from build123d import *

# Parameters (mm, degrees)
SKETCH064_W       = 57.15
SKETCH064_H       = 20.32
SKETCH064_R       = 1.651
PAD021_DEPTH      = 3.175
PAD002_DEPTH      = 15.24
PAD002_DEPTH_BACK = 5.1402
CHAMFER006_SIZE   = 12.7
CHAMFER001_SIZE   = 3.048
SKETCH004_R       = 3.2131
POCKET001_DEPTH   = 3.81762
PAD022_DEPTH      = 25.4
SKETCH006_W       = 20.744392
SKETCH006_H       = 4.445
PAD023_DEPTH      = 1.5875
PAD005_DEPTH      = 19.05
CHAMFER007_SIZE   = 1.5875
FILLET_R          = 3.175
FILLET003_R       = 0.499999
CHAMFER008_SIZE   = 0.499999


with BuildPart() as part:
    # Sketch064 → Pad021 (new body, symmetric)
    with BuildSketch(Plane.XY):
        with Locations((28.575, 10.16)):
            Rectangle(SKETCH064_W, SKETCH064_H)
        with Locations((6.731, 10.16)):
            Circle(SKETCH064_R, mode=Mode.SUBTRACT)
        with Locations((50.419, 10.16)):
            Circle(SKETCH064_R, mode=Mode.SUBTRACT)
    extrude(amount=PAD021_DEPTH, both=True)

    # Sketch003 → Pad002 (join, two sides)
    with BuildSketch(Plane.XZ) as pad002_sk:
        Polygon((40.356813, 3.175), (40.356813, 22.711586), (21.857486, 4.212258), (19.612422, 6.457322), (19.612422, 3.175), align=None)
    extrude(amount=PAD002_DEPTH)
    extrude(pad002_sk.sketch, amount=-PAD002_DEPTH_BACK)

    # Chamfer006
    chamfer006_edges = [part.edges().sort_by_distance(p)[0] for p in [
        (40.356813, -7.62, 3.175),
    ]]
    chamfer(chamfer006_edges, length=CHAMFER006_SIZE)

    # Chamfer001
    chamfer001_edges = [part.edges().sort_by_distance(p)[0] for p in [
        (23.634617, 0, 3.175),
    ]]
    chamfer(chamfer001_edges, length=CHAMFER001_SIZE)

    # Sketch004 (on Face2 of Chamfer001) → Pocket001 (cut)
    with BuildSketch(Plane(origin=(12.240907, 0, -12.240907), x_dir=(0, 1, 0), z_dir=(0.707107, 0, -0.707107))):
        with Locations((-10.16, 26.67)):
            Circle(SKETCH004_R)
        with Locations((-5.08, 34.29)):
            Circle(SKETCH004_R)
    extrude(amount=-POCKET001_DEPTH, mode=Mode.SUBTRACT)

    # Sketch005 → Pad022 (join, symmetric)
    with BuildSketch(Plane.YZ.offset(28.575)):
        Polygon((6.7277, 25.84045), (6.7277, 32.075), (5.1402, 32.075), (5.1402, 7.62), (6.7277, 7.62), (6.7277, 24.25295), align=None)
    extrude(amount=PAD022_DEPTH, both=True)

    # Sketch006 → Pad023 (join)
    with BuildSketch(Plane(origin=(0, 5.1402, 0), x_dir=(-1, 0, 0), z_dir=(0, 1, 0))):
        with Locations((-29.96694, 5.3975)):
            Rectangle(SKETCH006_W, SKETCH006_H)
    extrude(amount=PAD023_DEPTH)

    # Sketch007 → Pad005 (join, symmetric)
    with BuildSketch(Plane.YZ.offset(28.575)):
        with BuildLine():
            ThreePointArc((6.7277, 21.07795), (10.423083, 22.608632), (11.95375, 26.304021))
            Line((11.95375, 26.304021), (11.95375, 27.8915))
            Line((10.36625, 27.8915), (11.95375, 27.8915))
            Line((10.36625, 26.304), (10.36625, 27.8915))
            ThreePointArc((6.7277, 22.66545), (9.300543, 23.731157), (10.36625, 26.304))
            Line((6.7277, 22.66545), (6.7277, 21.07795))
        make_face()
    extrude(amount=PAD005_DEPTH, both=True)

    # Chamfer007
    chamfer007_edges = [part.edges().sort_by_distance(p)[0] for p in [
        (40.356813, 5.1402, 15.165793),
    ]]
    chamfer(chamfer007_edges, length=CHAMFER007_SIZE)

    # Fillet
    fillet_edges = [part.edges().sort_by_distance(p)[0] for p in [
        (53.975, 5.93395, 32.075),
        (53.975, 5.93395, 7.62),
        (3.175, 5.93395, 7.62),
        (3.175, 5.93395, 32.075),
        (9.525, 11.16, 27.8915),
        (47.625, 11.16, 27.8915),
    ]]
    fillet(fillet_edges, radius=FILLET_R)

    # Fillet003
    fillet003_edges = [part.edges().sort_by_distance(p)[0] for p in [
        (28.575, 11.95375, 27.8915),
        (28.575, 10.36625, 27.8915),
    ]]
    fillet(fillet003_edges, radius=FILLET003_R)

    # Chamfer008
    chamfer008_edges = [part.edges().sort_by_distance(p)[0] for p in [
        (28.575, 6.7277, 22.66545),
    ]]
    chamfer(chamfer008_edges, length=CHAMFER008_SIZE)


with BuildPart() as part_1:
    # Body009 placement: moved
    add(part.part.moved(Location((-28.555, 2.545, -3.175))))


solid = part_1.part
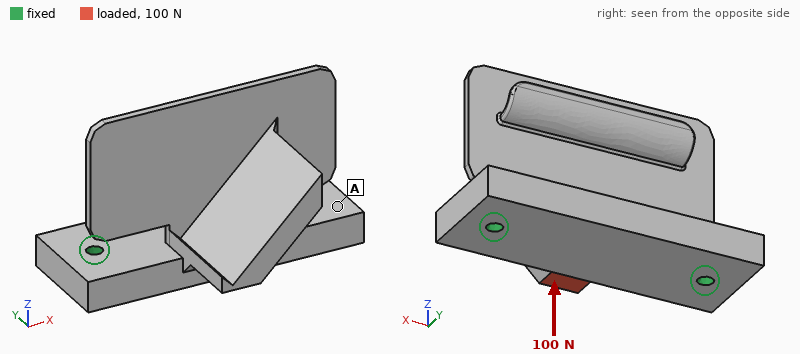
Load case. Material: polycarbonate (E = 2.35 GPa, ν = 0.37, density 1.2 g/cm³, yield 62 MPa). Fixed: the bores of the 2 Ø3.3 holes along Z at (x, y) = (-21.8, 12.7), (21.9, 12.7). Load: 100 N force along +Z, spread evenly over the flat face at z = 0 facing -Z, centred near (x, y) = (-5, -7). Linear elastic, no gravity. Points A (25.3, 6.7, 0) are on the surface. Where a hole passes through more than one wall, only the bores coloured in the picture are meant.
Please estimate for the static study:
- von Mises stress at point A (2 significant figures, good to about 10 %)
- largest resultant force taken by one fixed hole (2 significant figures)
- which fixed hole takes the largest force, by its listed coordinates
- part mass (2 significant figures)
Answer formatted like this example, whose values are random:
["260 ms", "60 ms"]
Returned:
["2.6 MPa", "69 N", "(-21.8, 12.7)", "15 g"]
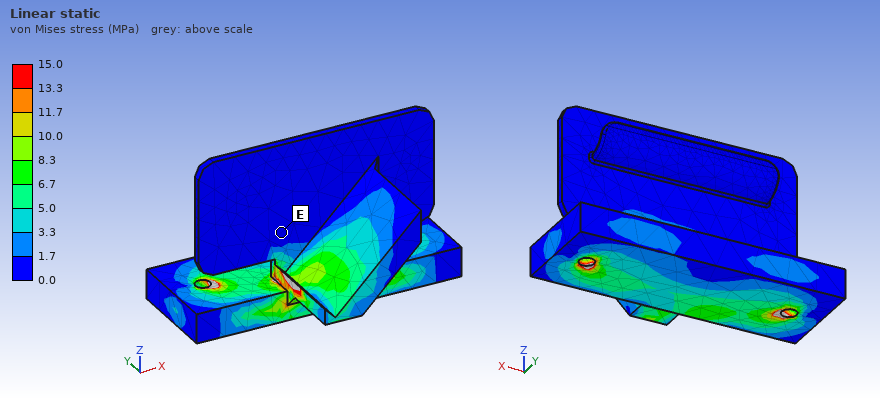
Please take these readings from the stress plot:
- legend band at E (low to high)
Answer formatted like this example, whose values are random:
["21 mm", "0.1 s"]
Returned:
["0.0 to 1.7 MPa"]
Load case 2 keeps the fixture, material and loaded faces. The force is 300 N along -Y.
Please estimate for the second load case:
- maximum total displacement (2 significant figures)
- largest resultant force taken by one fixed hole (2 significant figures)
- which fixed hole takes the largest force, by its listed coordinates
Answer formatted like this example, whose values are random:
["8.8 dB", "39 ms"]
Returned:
["0.40 mm", "190 N", "(-21.8, 12.7)"]
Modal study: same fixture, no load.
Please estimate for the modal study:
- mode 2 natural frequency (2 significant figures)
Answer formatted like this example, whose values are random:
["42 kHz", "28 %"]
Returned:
["1100 Hz"]
